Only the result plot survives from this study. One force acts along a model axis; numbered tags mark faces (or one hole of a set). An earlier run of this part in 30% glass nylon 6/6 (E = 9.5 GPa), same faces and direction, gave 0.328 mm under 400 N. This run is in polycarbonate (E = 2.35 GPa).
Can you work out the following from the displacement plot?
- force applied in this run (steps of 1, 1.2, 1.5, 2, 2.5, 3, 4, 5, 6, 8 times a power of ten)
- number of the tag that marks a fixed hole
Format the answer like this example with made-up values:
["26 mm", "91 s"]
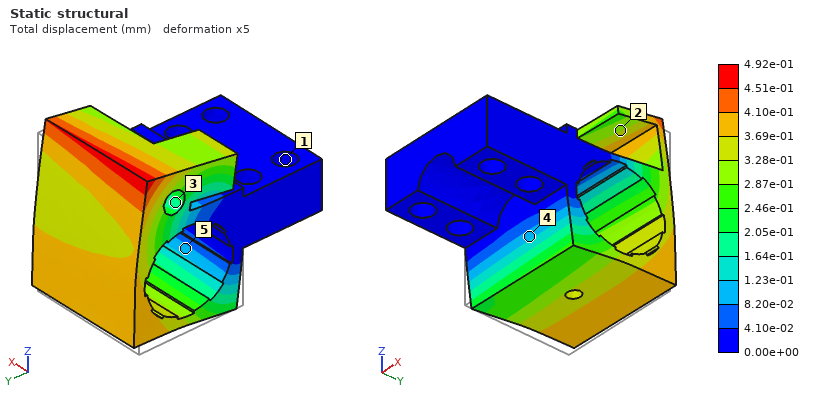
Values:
["150 N", "1"]
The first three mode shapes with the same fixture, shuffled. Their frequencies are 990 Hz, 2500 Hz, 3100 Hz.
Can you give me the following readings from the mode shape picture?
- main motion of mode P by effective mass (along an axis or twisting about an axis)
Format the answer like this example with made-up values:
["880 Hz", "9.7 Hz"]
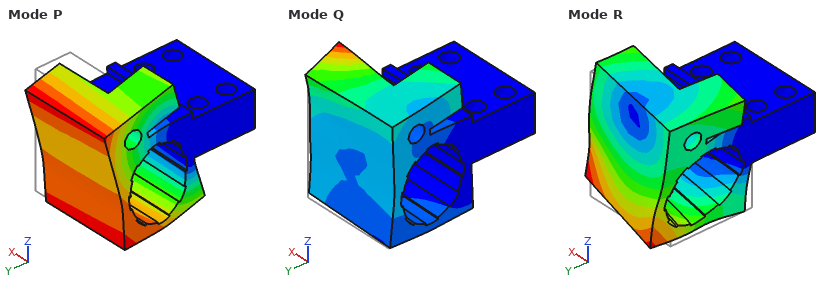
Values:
["along Z"]
